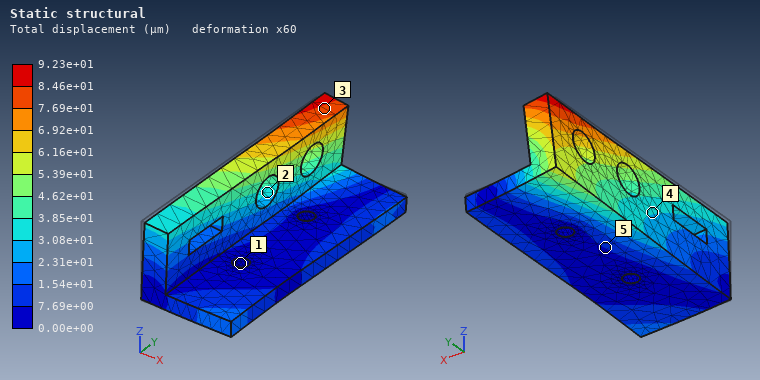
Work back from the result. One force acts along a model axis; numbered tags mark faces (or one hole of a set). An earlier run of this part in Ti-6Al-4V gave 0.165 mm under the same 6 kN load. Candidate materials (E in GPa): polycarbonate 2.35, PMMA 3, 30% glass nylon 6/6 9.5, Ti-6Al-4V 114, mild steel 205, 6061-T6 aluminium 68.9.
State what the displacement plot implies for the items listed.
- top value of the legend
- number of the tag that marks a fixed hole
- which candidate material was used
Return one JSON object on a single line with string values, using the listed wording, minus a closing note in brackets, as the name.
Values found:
{"top value of the legend": "9.23e+01 µm", "number of the tag that marks a fixed hole": "1", "which candidate material was used": "mild steel"}
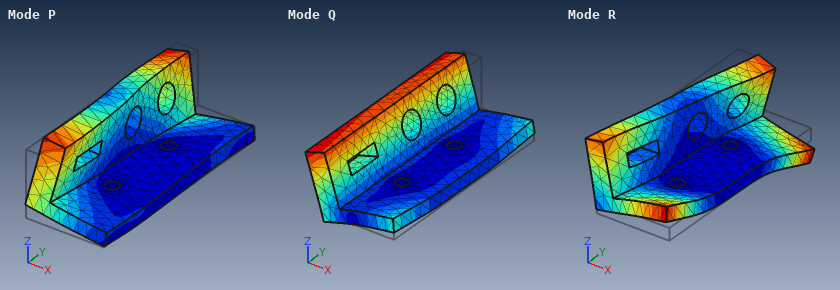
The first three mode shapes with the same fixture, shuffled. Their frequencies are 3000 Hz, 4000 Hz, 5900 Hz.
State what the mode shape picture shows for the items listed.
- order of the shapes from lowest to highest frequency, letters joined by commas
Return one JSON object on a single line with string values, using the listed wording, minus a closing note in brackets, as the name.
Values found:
{"order of the shapes from lowest to highest frequency, letters joined by commas": "Q, P, R"}
